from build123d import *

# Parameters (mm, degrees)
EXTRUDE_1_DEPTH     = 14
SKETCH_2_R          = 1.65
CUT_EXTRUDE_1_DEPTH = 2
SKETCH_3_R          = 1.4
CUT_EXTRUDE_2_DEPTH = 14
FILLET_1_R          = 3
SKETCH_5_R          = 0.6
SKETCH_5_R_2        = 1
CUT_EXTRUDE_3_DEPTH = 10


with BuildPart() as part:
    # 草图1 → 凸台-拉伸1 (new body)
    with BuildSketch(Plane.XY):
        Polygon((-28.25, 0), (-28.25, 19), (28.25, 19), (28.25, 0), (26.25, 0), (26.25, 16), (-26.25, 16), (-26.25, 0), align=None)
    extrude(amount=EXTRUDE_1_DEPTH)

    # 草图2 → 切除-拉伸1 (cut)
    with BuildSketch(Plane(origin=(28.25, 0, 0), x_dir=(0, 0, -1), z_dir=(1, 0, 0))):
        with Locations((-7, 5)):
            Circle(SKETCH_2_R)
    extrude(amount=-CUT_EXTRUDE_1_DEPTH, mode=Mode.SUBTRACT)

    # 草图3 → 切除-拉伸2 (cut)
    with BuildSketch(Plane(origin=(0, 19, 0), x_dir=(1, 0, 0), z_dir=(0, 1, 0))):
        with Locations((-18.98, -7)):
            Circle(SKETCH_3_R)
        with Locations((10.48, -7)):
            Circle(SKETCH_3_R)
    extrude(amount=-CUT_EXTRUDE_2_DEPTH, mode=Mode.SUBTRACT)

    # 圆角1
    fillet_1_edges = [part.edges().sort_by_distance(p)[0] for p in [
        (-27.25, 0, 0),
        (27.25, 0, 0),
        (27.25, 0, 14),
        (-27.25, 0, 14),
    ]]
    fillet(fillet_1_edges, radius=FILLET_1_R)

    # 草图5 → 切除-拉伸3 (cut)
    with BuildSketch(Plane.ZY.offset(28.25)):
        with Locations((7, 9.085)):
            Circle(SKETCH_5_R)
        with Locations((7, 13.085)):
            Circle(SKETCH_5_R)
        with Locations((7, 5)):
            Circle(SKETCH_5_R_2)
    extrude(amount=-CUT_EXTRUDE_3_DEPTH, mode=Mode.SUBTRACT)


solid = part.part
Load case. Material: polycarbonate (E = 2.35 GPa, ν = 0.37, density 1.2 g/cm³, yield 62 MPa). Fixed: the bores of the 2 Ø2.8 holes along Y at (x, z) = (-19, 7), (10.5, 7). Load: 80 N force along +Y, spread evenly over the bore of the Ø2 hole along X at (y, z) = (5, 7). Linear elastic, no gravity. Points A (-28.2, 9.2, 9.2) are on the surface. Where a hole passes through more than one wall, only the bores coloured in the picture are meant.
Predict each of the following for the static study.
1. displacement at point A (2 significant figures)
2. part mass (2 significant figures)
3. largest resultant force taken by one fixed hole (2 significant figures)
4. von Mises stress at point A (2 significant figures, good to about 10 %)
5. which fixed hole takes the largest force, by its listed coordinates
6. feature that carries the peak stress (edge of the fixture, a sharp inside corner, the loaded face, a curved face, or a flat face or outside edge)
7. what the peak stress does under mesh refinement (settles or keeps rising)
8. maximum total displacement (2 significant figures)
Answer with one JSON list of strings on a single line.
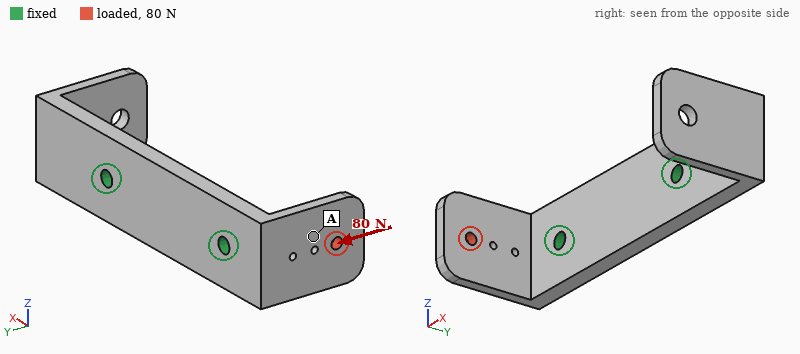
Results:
["0.41 mm", "3.8 g", "83 N", "4.0 MPa", "(-19, 7)", "edge of the fixture", "keeps rising", "0.70 mm"]
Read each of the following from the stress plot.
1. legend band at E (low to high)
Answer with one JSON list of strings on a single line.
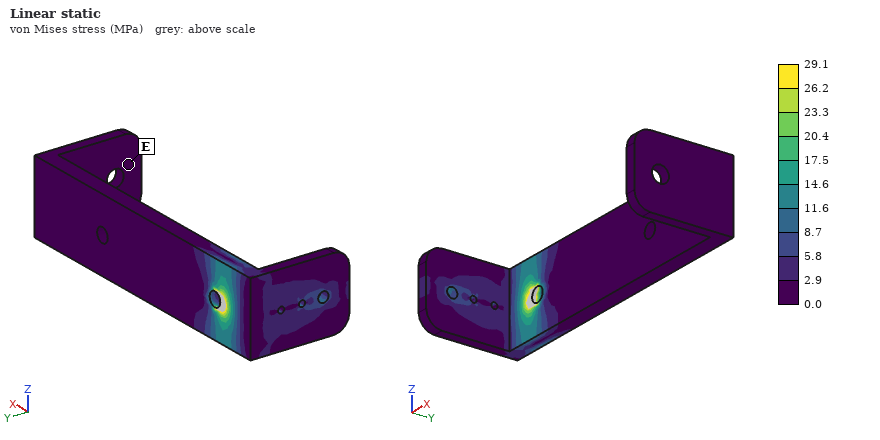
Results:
["0.0 to 2.9 MPa"]
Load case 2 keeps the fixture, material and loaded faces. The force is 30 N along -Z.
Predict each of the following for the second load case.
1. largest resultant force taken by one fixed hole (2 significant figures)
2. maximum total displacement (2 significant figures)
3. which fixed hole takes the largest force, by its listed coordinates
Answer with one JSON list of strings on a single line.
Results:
["36 N", "0.56 mm", "(-19, 7)"]
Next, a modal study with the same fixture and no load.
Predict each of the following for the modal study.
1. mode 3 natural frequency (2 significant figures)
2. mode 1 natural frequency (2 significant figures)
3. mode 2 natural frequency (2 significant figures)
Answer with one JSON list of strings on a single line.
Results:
["1400 Hz", "920 Hz", "1300 Hz"]
